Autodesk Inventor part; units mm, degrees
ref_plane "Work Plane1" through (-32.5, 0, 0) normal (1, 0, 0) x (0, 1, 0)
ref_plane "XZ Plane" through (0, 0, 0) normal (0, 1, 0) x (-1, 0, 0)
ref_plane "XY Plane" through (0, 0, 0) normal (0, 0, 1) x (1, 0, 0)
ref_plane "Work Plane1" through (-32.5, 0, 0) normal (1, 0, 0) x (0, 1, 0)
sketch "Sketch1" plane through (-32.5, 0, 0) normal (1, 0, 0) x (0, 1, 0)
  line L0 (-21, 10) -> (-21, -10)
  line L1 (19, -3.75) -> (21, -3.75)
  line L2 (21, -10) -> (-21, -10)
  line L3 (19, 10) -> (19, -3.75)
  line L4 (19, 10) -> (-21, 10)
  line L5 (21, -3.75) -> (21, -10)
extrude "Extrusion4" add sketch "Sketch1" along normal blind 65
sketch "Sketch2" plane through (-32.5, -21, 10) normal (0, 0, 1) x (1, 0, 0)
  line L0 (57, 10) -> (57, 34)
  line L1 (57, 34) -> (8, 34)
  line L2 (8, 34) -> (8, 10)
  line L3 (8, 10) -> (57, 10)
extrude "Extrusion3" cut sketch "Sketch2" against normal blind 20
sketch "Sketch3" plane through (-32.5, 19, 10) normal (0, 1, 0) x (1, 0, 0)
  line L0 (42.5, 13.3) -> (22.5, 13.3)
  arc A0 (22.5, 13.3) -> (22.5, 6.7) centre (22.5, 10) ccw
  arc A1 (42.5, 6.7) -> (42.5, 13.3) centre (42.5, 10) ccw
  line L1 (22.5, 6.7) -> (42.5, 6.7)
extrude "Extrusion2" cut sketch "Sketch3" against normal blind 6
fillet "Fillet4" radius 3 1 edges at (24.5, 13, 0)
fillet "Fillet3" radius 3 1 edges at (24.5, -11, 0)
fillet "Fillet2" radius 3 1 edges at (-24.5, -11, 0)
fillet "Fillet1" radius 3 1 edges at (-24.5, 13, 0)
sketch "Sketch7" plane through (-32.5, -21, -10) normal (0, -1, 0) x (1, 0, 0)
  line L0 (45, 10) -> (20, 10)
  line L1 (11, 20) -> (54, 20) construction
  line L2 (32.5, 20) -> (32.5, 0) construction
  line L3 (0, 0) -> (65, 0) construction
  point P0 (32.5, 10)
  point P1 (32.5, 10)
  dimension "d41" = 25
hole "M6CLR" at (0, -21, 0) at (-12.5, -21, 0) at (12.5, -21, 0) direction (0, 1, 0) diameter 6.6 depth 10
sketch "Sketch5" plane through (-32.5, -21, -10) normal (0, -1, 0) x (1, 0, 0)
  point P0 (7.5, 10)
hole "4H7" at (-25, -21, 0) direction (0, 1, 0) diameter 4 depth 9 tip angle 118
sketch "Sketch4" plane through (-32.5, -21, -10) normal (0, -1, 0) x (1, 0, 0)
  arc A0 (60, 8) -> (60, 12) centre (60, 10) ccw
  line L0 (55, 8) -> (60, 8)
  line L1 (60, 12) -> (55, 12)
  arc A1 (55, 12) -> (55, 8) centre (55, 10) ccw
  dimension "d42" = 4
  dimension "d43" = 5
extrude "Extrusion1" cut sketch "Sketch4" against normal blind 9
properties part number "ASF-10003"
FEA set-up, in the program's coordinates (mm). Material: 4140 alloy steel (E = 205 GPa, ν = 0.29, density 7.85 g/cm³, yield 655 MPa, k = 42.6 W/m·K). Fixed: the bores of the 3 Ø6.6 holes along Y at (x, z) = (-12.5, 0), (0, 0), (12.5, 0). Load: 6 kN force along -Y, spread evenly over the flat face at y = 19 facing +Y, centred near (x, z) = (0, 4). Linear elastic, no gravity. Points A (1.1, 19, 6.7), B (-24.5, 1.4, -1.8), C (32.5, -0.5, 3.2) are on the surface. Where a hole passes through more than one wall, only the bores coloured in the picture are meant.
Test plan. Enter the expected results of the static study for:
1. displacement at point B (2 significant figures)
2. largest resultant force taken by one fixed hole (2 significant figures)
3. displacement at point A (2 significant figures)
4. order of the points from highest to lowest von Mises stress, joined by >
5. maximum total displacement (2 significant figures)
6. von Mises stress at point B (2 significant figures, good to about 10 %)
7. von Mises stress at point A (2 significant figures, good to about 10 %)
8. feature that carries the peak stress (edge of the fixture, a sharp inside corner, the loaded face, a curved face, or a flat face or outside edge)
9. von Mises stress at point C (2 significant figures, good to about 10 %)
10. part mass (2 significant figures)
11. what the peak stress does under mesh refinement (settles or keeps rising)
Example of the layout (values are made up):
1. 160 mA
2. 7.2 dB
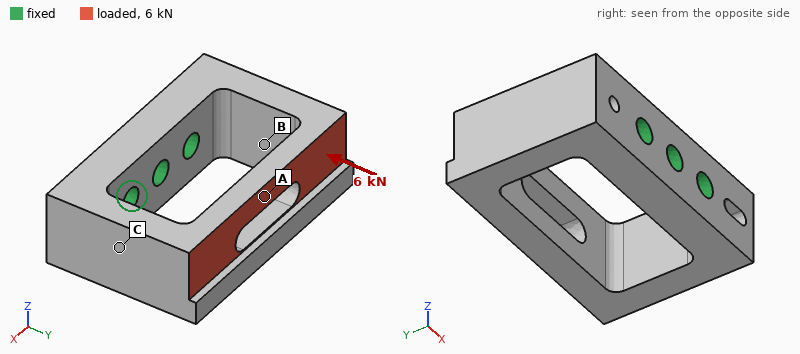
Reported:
1. 16 µm
2. 3.4 kN
3. 70 µm
4. A > B > C
5. 75 µm
6. 77 MPa
7. 140 MPa
8. edge of the fixture
9. 36 MPa
10. 210 g
11. keeps rising
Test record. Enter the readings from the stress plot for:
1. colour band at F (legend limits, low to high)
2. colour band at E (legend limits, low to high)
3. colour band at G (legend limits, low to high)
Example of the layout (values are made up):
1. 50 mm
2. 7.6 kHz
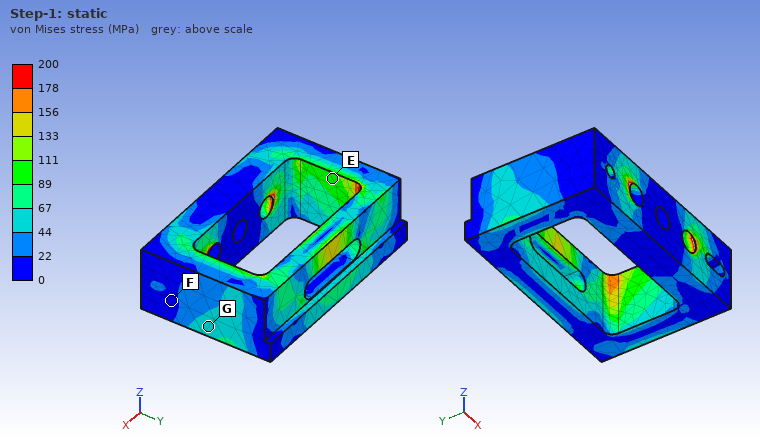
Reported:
1. 0 to 22 MPa
2. 89 to 111 MPa
3. 44 to 67 MPa
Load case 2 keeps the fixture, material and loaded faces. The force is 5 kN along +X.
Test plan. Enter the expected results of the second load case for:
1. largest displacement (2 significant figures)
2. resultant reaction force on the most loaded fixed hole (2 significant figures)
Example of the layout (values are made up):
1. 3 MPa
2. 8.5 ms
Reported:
1. 0.14 mm
2. 3.3 kN
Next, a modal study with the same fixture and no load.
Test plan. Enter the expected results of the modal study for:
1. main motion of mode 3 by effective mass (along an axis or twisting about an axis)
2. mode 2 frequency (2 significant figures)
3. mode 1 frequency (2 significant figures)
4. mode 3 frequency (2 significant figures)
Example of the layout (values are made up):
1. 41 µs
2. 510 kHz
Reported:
1. twisting about Y
2. 3600 Hz
3. 3600 Hz
4. 5400 Hz
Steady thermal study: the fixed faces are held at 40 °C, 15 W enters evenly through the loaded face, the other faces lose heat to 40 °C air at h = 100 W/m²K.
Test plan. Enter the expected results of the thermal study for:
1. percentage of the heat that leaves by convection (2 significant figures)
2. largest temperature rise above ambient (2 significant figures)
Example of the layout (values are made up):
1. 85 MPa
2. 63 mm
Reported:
1. 66 %
2. 32 K
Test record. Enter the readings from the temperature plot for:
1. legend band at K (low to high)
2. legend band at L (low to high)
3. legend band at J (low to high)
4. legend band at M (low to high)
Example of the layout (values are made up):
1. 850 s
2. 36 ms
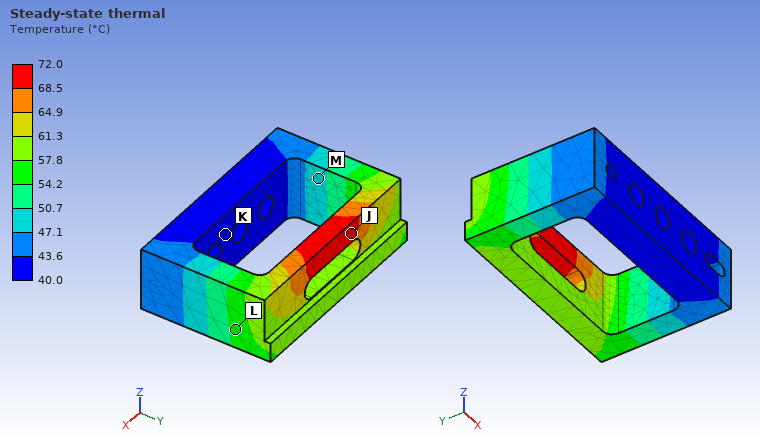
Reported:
1. 40.0 to 43.6 °C
2. 54.2 to 57.8 °C
3. 68.5 to 72.0 °C
4. 47.1 to 50.7 °C
